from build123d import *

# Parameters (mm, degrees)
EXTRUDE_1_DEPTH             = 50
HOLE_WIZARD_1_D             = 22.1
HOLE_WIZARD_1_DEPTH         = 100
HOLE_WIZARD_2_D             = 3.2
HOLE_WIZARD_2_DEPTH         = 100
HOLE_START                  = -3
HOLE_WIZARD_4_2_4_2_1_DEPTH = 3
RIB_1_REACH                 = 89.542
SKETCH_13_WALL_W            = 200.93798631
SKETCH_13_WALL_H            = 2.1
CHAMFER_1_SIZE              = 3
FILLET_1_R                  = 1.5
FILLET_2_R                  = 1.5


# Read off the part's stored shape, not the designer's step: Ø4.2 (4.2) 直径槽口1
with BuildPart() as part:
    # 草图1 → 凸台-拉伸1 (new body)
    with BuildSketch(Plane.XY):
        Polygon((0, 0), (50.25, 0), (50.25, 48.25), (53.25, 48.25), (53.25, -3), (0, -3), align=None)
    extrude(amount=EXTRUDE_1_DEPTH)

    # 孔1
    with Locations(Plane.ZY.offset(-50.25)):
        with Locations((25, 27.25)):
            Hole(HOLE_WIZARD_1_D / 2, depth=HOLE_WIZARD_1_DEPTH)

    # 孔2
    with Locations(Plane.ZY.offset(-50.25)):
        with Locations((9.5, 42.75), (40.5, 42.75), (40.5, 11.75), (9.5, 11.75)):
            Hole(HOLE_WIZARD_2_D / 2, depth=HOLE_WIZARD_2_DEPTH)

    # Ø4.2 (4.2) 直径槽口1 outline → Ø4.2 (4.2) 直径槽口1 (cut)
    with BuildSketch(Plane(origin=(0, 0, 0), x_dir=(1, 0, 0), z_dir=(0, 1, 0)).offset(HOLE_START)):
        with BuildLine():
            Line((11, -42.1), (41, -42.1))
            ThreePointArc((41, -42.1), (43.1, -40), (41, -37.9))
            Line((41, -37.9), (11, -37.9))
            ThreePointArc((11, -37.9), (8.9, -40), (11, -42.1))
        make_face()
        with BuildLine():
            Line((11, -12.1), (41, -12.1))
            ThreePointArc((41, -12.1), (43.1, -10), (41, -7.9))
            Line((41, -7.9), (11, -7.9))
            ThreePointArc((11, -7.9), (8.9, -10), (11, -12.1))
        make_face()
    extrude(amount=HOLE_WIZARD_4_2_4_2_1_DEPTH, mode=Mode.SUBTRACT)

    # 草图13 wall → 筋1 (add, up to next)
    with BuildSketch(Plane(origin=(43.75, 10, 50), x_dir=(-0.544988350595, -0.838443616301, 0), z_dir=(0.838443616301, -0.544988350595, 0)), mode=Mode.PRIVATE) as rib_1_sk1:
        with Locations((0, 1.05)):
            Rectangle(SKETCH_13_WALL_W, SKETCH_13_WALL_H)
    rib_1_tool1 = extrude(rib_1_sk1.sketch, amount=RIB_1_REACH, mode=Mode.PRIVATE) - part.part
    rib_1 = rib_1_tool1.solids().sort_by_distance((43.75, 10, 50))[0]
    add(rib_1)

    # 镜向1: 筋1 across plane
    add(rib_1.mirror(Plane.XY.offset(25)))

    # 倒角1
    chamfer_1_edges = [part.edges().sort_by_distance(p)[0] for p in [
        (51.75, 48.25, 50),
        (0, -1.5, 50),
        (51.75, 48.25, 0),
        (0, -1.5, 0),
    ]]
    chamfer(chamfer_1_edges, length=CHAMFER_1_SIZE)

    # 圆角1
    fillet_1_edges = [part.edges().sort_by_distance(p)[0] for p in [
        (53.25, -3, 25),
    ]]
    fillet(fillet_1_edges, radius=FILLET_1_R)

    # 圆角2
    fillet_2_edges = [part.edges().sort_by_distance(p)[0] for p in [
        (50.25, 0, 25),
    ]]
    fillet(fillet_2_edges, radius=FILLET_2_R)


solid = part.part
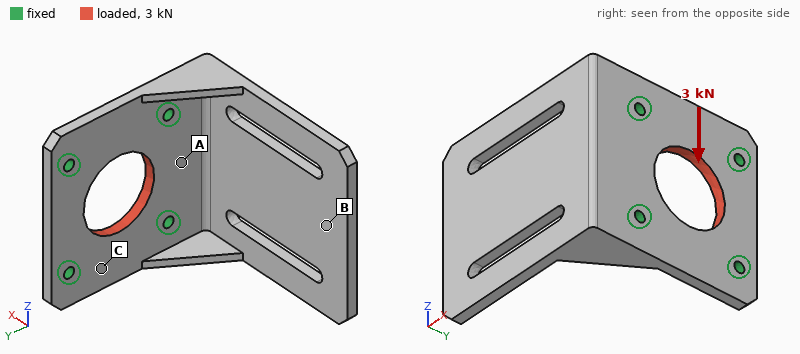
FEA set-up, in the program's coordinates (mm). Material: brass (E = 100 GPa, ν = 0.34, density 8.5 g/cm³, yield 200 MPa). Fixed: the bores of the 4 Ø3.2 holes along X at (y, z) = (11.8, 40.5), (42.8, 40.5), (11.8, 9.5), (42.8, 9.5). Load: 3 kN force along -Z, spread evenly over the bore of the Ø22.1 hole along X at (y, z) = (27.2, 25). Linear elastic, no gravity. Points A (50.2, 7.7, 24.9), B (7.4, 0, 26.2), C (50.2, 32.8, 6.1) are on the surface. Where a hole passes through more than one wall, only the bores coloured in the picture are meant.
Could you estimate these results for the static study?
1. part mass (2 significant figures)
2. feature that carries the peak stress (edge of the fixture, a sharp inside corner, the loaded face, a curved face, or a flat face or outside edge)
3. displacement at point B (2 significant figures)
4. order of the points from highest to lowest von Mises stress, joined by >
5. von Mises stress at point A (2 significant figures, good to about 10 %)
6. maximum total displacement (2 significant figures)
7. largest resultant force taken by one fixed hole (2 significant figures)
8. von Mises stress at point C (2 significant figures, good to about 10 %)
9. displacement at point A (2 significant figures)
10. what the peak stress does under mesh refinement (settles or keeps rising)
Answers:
120 g
edge of the fixture
0.92 µm
C > A > B
7.0 MPa
4.9 µm
780 N
12 MPa
0.99 µm
keeps rising
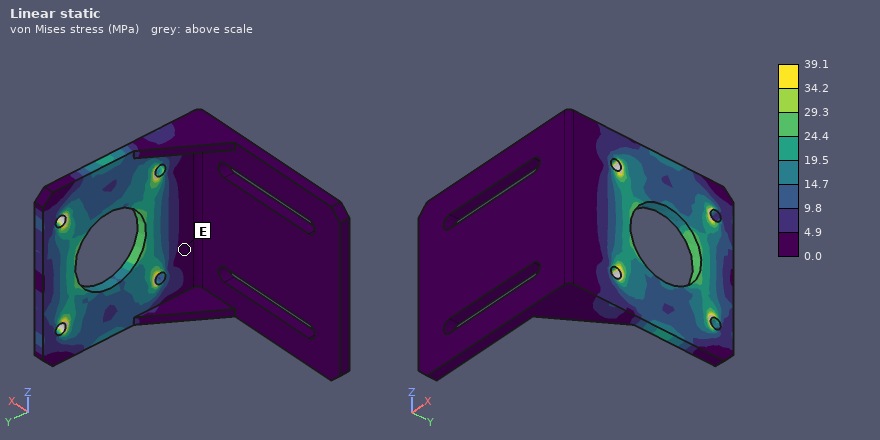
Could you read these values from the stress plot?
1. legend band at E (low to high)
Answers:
0.0 to 4.9 MPa
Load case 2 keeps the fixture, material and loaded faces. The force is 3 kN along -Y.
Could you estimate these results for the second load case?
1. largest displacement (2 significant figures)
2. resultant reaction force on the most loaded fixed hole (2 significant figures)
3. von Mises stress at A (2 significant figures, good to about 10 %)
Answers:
6.5 µm
780 N
8.1 MPa
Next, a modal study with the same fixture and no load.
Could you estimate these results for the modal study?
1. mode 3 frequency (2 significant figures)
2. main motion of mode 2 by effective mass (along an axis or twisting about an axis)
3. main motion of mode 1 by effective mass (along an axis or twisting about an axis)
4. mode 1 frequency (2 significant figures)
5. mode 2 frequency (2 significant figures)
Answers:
2100 Hz
along Z
along Y
610 Hz
1400 Hz
